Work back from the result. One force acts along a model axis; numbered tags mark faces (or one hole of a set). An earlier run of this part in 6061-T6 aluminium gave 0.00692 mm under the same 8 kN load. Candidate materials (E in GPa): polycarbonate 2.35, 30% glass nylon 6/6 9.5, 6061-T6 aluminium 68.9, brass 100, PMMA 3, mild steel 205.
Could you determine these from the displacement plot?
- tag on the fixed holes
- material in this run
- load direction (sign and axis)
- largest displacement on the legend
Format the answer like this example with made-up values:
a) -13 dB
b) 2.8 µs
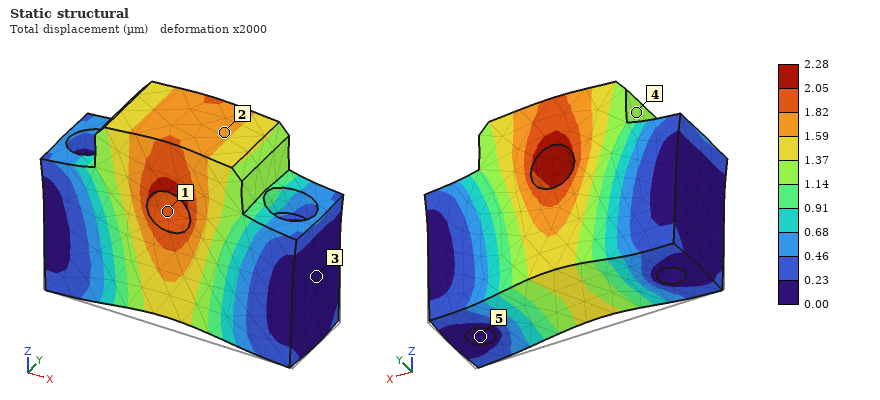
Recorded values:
a) 5
b) mild steel
c) +Z
d) 2.28 µm
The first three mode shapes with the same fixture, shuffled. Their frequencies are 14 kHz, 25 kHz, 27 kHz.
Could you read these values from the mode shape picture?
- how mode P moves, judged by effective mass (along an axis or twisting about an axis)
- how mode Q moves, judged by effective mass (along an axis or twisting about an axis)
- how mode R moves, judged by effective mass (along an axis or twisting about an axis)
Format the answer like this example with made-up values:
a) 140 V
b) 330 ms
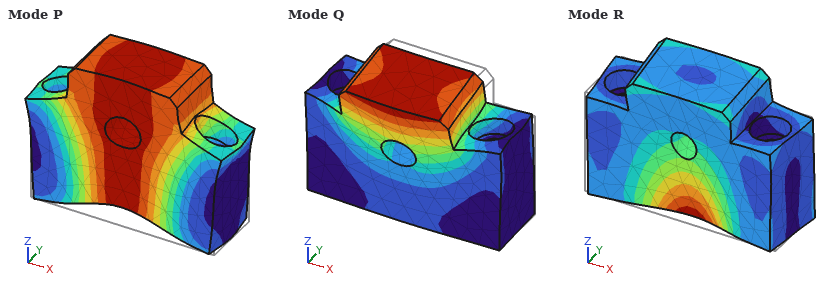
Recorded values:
a) along Z
b) along Y
c) along Y
